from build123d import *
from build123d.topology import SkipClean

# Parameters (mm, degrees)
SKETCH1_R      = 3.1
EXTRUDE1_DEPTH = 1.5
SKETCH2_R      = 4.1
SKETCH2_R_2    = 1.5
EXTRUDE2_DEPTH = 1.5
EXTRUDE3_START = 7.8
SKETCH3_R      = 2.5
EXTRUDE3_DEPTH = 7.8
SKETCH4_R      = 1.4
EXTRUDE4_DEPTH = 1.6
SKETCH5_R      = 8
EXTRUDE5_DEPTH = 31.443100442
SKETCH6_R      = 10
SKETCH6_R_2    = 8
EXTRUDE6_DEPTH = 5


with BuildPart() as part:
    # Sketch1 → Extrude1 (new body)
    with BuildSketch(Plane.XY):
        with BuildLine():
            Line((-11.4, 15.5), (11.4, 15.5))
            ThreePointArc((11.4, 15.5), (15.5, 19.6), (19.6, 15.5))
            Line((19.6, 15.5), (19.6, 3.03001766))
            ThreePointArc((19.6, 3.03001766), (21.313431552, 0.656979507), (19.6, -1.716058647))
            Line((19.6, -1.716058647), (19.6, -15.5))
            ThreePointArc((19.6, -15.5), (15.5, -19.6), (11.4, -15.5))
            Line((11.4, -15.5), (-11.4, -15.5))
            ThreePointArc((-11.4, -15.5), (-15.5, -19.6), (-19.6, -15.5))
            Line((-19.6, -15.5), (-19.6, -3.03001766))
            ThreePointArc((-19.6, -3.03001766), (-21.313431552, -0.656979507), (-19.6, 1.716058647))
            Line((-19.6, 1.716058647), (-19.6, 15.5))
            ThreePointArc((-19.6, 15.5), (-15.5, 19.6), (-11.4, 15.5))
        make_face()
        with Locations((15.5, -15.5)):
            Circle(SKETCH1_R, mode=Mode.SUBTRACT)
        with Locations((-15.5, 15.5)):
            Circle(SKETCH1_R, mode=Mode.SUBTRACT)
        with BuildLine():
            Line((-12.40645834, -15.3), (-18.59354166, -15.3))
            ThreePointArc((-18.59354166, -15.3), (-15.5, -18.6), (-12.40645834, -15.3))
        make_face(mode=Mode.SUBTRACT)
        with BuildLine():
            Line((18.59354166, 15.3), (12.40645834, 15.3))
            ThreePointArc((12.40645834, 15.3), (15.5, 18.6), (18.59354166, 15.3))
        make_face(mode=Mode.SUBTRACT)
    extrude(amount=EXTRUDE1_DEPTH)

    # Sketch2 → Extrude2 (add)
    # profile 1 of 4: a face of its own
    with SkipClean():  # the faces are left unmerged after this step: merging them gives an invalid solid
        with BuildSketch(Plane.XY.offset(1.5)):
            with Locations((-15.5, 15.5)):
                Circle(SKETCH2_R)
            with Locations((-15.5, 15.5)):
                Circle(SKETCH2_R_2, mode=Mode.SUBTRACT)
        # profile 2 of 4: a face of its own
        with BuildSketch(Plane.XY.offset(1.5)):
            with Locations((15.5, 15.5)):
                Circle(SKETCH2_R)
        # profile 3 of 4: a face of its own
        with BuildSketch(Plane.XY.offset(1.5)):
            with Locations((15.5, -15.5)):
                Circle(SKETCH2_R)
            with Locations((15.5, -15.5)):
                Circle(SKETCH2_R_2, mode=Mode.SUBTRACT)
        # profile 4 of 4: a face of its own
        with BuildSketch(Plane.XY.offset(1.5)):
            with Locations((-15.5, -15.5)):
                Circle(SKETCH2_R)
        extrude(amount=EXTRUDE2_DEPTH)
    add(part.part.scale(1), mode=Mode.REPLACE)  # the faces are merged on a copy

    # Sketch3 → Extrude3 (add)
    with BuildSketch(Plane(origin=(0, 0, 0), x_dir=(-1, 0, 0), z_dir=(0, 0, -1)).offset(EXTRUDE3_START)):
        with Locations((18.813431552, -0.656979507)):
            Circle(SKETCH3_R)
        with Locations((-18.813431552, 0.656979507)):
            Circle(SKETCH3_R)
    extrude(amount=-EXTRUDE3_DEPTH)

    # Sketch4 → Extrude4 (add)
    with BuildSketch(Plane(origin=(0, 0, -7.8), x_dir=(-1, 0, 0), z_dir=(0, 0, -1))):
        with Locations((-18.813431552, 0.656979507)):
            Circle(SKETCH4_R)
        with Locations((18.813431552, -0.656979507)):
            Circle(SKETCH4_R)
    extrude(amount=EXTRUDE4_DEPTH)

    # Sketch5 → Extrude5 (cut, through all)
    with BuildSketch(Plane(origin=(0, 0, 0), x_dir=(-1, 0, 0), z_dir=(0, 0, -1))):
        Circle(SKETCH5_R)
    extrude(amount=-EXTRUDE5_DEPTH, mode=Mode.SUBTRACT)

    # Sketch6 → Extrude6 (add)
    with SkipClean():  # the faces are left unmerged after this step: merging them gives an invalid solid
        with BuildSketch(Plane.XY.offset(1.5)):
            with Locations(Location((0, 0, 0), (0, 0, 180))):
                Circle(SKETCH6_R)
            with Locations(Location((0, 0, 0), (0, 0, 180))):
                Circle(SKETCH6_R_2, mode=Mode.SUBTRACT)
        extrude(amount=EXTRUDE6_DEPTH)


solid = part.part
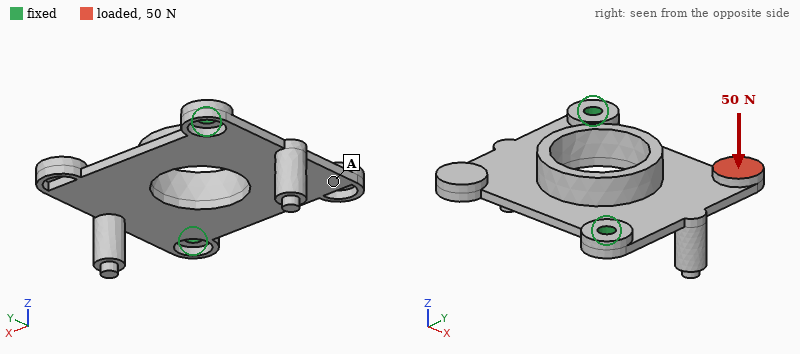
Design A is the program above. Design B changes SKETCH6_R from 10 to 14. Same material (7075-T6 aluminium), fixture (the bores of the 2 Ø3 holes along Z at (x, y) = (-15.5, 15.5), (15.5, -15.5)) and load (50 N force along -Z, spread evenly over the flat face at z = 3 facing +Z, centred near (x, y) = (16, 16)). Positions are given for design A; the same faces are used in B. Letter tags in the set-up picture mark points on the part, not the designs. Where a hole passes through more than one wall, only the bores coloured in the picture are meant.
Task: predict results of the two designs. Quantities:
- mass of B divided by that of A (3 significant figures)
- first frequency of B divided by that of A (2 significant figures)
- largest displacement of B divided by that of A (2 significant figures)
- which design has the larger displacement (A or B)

1.55
1.1
0.55
A
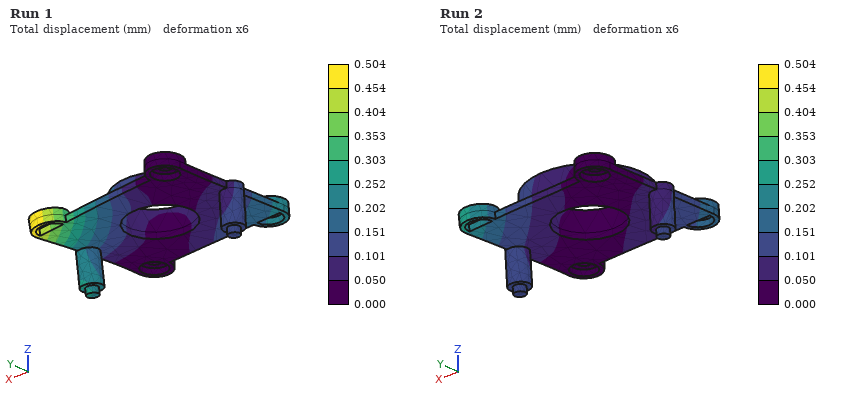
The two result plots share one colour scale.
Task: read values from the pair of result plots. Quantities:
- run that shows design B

Run 2
